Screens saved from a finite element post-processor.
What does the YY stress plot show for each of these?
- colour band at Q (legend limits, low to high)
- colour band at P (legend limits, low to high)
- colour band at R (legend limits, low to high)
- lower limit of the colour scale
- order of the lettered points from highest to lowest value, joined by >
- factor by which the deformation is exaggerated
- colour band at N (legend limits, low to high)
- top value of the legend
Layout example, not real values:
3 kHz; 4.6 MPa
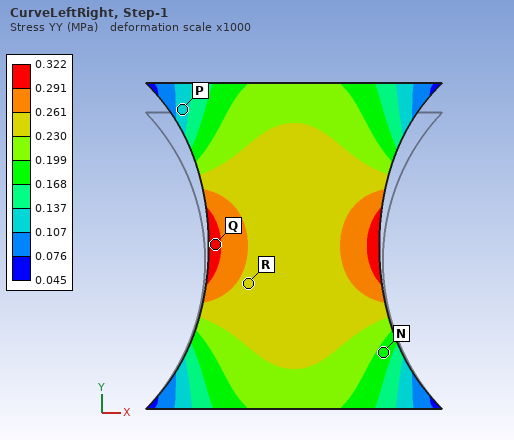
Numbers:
0.291 to 0.322 MPa; 0.107 to 0.137 MPa; 0.230 to 0.261 MPa; 0.045 MPa; Q > R > N > P; 1000; 0.168 to 0.199 MPa; 0.322 MPa
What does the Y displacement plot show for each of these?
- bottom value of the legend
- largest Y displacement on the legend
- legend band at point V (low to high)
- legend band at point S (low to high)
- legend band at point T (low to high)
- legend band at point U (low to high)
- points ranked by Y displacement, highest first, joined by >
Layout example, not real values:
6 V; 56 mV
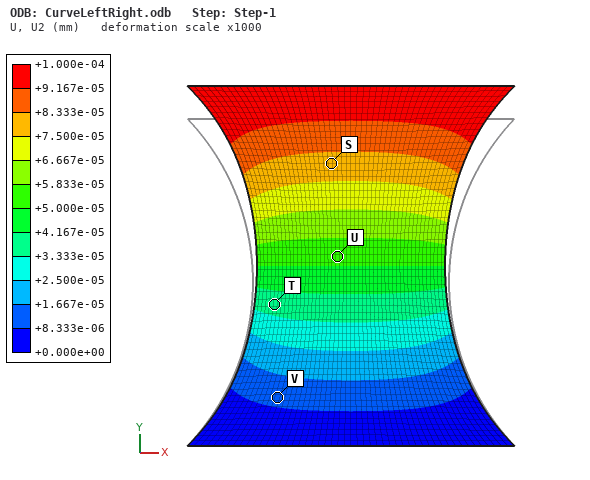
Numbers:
+0.000e+00 mm; +1.000e-04 mm; +8.333e-06 to +1.667e-05 mm; +7.500e-05 to +8.333e-05 mm; +3.333e-05 to +4.167e-05 mm; +5.000e-05 to +5.833e-05 mm; S > U > T > V
